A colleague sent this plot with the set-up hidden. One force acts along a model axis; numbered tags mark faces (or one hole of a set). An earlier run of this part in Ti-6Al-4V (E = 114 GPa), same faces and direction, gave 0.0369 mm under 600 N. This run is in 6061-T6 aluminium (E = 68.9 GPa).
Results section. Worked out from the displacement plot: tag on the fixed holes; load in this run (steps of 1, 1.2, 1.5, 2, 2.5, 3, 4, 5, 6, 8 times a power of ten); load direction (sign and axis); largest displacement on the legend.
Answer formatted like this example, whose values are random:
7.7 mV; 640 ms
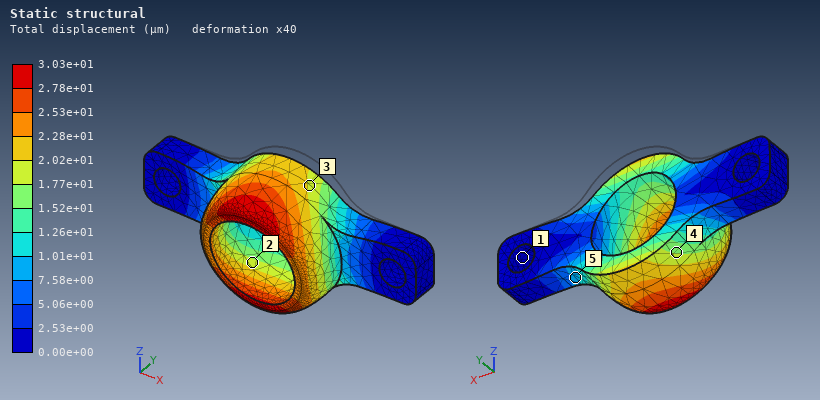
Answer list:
1; 300 N; -Z; 3.03e+01 µm
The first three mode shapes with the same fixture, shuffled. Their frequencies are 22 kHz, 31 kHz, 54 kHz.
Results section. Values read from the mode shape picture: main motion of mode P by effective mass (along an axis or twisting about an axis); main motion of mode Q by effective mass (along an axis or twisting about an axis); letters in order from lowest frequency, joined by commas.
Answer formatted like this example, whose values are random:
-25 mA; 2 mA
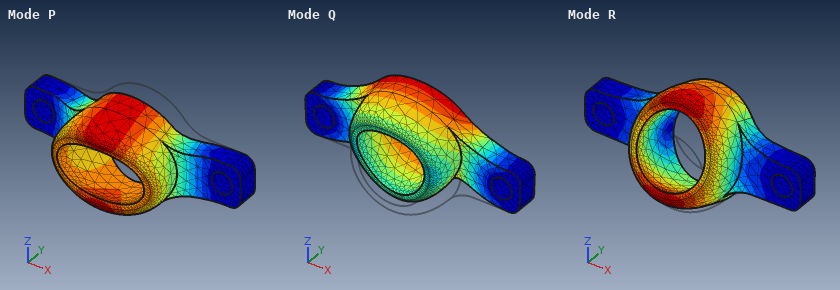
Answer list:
along Y; along Z; R, P, Q
